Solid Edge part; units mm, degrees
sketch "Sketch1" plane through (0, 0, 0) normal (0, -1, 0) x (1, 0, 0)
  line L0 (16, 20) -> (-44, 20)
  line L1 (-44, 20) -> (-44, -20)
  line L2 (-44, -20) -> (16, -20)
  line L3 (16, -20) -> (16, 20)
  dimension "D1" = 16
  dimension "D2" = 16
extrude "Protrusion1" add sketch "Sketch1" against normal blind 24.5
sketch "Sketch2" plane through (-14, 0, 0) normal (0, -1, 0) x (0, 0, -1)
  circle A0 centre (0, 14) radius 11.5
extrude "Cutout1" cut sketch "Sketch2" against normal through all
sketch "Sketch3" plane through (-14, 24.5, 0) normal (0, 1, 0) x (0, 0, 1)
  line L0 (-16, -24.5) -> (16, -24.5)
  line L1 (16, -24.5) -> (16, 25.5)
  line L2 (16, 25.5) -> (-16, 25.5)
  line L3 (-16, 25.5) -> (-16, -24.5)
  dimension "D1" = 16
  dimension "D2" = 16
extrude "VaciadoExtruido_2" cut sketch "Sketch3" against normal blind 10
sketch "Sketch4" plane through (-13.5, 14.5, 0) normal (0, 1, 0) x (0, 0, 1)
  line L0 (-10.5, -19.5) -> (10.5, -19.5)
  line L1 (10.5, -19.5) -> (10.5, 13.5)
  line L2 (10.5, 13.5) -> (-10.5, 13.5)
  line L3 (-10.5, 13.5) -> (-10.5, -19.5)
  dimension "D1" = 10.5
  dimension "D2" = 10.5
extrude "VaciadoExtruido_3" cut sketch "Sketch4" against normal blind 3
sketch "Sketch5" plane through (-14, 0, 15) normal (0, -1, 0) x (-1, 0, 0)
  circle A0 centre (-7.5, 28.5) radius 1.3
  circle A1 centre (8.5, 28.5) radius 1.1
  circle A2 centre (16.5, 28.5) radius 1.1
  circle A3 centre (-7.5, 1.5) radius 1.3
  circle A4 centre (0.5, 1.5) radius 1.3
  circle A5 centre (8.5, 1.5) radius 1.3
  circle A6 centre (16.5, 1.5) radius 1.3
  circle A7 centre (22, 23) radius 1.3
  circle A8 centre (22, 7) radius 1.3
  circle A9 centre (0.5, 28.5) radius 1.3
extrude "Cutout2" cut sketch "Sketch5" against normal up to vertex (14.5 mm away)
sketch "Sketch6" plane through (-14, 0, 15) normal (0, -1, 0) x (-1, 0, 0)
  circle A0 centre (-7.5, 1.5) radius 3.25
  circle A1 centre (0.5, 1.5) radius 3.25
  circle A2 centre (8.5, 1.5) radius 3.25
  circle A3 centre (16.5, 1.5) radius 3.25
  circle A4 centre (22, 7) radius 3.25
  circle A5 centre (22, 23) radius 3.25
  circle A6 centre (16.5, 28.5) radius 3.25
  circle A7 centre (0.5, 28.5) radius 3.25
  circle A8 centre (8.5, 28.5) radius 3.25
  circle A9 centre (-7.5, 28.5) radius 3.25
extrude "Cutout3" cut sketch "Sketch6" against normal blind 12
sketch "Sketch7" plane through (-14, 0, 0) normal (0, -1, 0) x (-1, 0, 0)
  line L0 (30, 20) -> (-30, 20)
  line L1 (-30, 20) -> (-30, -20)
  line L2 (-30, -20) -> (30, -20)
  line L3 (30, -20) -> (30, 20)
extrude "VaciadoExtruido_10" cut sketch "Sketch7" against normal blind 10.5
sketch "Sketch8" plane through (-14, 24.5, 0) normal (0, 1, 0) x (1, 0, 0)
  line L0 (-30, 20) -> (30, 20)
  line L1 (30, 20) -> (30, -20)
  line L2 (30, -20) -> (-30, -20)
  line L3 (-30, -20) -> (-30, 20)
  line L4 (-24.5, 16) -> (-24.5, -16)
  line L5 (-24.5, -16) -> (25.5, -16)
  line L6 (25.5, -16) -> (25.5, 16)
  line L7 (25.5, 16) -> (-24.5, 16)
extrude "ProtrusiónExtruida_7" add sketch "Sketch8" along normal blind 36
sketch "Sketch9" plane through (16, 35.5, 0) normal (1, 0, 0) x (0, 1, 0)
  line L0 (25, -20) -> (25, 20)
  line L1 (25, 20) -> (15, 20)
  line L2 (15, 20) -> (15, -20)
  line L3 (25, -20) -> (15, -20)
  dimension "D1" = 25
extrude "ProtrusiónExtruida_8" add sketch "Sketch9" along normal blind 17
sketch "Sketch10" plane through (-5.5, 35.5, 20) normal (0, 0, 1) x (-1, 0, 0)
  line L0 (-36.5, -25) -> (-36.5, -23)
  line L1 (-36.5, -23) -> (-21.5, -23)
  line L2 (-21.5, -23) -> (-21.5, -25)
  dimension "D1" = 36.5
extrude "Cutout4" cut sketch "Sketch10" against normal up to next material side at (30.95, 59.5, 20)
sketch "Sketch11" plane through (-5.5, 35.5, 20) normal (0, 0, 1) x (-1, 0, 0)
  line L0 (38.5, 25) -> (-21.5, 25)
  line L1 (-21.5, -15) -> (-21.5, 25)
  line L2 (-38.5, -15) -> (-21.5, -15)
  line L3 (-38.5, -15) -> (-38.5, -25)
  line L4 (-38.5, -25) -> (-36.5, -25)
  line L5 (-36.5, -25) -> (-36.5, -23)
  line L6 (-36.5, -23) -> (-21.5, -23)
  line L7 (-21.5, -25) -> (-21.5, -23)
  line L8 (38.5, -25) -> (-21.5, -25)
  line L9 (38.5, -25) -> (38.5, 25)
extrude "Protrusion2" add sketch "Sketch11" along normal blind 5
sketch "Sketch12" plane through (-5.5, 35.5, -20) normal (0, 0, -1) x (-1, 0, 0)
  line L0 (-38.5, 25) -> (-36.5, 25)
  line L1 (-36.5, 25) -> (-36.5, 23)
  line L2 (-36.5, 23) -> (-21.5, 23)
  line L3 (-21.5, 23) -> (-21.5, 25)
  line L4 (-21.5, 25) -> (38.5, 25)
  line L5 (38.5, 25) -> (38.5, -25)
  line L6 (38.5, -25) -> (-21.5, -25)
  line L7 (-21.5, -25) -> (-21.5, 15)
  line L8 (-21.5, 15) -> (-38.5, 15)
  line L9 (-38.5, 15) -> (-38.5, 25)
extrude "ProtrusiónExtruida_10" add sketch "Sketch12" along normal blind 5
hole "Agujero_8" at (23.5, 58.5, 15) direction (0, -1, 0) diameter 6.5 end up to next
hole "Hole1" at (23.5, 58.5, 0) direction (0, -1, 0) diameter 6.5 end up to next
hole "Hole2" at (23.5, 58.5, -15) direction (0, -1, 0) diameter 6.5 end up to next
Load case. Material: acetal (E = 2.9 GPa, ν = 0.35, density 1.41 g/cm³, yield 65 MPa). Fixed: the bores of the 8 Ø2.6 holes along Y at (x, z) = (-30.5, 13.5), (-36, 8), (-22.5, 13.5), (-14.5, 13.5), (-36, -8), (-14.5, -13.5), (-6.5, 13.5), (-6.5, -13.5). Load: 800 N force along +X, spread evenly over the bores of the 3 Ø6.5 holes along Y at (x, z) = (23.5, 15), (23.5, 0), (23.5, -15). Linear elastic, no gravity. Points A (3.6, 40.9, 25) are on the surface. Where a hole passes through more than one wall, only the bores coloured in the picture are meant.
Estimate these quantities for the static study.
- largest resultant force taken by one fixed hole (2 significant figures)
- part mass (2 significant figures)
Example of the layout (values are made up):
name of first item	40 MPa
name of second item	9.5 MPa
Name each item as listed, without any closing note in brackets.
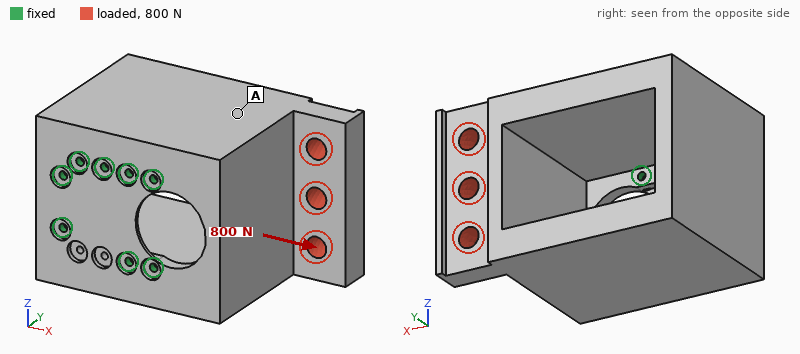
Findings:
largest resultant force taken by one fixed hole	520 N
part mass	110 g
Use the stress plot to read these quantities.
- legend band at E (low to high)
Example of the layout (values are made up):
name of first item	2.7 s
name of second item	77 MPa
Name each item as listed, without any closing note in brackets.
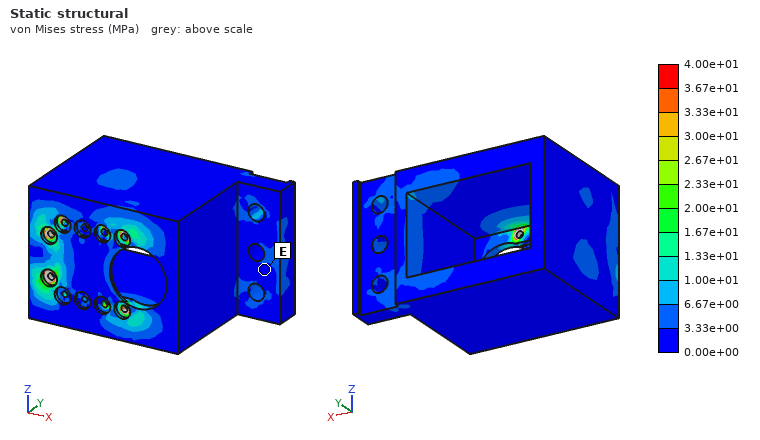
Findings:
legend band at E	0.00e+00 to 3.33e+00 MPa
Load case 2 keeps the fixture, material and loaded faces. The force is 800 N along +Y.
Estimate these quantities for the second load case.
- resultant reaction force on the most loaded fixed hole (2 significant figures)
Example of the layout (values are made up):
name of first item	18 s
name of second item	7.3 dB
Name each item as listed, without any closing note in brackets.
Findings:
resultant reaction force on the most loaded fixed hole	620 N
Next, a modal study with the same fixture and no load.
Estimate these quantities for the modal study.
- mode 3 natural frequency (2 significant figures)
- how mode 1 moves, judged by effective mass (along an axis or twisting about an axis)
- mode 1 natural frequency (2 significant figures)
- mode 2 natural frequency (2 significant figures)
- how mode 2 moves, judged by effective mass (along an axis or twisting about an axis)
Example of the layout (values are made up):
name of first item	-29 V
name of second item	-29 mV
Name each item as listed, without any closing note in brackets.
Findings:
mode 3 natural frequency	1500 Hz
how mode 1 moves, judged by effective mass	along Z
mode 1 natural frequency	670 Hz
mode 2 natural frequency	770 Hz
how mode 2 moves, judged by effective mass	along X
